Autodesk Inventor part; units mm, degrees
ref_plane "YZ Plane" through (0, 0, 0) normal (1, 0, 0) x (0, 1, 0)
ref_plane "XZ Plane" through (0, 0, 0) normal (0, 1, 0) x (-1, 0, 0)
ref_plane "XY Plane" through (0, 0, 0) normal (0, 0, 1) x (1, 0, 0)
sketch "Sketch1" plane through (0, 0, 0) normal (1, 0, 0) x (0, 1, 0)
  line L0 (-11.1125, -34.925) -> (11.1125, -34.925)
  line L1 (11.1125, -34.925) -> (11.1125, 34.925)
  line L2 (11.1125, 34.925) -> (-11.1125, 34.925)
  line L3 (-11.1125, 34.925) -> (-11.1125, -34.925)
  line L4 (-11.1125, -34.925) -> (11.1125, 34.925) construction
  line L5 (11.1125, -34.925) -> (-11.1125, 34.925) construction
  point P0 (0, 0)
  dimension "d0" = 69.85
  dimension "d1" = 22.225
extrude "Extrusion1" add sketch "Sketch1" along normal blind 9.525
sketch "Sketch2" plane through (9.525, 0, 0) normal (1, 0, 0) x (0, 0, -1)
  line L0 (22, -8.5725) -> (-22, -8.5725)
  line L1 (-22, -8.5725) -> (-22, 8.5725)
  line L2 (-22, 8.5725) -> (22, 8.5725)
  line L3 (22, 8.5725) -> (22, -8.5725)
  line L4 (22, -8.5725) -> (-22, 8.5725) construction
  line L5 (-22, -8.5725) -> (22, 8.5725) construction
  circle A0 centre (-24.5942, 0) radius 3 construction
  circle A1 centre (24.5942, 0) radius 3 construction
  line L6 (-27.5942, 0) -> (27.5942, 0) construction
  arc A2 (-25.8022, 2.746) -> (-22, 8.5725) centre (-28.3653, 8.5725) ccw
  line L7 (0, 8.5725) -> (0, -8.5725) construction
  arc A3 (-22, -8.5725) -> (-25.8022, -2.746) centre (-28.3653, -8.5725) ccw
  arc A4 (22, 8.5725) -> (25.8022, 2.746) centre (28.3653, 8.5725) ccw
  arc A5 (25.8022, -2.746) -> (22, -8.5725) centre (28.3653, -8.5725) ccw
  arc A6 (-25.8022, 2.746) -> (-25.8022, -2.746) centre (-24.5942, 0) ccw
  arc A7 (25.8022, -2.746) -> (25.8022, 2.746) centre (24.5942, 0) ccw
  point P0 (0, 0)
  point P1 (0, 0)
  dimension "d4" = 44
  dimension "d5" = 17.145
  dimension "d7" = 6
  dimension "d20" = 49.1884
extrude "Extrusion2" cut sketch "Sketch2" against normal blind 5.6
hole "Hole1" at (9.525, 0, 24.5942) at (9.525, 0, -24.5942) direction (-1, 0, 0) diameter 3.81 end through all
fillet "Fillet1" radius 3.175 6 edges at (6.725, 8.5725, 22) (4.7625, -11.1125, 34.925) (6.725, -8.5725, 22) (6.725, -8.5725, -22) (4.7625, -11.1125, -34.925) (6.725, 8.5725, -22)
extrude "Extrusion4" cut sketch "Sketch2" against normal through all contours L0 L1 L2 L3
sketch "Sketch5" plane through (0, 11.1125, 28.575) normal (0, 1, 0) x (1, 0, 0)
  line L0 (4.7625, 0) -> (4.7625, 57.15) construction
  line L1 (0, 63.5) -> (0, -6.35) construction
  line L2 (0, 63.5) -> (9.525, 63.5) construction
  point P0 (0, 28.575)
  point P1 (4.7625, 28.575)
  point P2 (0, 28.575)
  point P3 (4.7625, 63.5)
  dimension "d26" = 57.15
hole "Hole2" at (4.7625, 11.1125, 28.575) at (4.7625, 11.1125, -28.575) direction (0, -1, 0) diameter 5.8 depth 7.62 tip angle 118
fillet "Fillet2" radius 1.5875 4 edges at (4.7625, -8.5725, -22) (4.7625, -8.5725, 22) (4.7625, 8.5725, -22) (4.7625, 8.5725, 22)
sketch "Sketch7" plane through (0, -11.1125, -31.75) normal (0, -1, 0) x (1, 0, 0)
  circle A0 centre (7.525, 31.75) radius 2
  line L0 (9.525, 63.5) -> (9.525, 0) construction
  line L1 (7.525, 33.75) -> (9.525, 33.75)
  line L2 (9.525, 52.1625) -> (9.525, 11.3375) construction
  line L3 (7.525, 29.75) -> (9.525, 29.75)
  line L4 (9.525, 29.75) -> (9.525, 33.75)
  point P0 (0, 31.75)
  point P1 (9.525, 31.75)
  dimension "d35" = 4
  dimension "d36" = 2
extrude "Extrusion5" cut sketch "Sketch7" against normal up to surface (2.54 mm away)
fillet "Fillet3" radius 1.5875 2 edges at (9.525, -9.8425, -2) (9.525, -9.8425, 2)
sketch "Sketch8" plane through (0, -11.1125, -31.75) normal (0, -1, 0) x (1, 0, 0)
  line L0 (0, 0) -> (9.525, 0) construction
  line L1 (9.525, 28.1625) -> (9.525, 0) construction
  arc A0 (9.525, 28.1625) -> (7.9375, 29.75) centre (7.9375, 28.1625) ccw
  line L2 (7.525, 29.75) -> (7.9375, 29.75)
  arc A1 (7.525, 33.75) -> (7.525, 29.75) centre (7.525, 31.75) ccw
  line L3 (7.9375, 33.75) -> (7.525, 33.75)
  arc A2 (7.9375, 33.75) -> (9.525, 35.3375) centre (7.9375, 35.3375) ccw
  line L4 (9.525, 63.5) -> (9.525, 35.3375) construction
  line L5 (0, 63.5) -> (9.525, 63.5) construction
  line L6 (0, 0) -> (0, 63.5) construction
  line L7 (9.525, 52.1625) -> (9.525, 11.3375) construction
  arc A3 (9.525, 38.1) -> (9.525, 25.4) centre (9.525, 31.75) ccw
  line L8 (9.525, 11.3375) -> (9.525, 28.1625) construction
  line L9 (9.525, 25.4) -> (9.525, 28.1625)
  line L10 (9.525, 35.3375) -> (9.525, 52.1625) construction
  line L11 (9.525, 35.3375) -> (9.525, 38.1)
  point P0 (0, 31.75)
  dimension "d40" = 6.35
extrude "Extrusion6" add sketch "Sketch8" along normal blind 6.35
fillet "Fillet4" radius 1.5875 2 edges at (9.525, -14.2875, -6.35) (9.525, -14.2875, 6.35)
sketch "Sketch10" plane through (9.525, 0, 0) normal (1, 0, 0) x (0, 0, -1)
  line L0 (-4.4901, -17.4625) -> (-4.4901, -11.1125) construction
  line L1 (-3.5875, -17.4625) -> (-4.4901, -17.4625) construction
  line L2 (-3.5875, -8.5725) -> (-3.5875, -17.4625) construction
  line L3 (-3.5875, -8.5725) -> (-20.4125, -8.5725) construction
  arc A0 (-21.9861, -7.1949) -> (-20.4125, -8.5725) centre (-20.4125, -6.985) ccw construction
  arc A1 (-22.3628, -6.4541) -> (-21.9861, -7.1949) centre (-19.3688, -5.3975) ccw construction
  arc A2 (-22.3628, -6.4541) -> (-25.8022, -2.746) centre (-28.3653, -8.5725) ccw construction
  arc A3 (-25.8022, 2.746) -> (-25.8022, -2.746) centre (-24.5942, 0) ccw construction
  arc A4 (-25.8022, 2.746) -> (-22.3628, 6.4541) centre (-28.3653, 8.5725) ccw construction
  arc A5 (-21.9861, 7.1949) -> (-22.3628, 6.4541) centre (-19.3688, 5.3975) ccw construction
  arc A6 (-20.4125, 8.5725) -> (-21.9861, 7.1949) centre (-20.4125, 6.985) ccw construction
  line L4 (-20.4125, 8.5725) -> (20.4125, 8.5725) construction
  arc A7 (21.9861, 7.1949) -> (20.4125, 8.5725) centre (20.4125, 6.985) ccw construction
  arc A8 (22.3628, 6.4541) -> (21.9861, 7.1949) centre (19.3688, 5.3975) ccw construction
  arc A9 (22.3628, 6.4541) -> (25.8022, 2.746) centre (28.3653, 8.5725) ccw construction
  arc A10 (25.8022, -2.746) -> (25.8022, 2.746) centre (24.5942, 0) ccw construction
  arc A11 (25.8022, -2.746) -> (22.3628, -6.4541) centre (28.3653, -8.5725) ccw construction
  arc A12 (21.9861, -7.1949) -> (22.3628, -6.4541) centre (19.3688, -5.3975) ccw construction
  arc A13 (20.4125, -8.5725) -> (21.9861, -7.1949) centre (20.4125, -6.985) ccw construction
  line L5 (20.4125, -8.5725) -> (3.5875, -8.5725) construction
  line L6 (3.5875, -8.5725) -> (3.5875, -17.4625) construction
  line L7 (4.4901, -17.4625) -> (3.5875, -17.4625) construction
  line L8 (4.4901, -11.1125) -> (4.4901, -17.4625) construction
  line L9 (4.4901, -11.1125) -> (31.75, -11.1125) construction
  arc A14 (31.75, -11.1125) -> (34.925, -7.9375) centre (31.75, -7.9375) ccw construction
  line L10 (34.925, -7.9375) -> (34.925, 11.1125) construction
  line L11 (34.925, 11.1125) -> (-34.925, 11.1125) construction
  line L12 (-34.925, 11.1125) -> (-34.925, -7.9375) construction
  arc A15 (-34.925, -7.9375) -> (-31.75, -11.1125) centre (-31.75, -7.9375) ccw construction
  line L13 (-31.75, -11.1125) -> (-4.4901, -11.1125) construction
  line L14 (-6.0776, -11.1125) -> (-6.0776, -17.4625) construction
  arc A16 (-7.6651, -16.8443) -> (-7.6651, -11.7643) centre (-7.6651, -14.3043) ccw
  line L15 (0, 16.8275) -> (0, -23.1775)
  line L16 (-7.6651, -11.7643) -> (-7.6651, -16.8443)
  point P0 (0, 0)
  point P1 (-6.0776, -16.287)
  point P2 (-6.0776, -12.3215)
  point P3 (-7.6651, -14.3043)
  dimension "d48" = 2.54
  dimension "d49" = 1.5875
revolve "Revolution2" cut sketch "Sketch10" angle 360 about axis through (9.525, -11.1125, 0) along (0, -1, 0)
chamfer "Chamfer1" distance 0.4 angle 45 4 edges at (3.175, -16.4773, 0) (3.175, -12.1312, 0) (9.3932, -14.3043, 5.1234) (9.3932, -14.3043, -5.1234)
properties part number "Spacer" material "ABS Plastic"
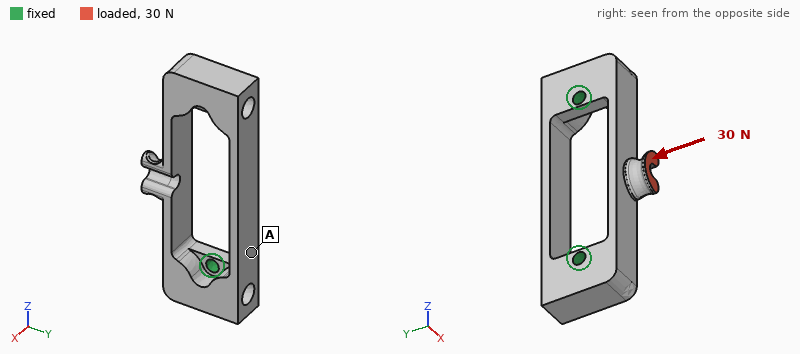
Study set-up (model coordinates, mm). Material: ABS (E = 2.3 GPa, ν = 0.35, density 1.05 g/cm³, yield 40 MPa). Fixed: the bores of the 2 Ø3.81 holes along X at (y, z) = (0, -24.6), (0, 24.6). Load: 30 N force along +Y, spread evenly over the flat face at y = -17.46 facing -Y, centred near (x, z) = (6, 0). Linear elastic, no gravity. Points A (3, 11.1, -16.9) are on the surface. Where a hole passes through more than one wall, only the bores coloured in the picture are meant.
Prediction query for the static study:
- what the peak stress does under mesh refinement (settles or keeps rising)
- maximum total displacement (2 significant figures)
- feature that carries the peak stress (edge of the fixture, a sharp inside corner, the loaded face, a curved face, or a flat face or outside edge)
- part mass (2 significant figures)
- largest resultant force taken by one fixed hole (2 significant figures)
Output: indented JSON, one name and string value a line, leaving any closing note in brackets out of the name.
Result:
{
  "what the peak stress does under mesh refinement": "keeps rising",
  "maximum total displacement": "0.40 mm",
  "feature that carries the peak stress": "a sharp inside corner",
  "part mass": "7.1 g",
  "largest resultant force taken by one fixed hole": "21 N"
}
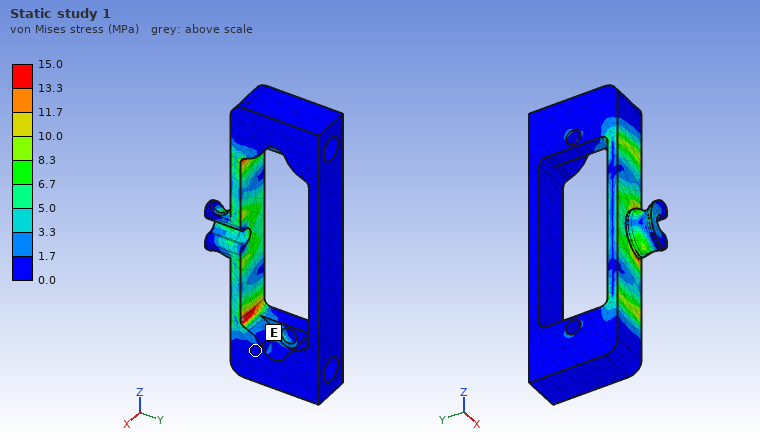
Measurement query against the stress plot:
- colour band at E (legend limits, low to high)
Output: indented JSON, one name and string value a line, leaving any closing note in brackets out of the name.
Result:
{
  "colour band at E": "0.0 to 1.7 MPa"
}
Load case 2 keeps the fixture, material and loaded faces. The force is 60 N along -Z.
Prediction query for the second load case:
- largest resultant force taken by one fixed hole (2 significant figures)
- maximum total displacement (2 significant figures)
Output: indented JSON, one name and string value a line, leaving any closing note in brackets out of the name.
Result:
{
  "largest resultant force taken by one fixed hole": "34 N",
  "maximum total displacement": "0.29 mm"
}
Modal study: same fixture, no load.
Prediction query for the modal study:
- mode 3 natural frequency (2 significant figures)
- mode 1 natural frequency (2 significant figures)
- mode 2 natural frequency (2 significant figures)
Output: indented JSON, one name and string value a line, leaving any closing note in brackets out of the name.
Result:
{
  "mode 3 natural frequency": "2200 Hz",
  "mode 1 natural frequency": "1700 Hz",
  "mode 2 natural frequency": "1800 Hz"
}
